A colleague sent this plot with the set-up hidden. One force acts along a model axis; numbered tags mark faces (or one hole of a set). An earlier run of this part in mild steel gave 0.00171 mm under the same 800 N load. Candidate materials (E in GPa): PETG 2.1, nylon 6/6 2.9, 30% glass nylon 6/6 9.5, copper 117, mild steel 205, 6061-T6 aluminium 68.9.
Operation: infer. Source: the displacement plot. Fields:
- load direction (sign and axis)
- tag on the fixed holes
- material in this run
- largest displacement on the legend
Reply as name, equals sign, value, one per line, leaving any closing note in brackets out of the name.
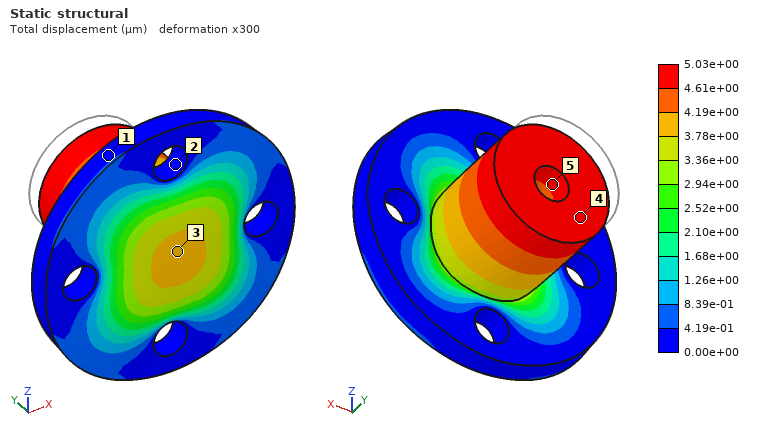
load direction = -Y
tag on the fixed holes = 2
material in this run = 6061-T6 aluminium
largest displacement on the legend = 5.03e+00 µm
